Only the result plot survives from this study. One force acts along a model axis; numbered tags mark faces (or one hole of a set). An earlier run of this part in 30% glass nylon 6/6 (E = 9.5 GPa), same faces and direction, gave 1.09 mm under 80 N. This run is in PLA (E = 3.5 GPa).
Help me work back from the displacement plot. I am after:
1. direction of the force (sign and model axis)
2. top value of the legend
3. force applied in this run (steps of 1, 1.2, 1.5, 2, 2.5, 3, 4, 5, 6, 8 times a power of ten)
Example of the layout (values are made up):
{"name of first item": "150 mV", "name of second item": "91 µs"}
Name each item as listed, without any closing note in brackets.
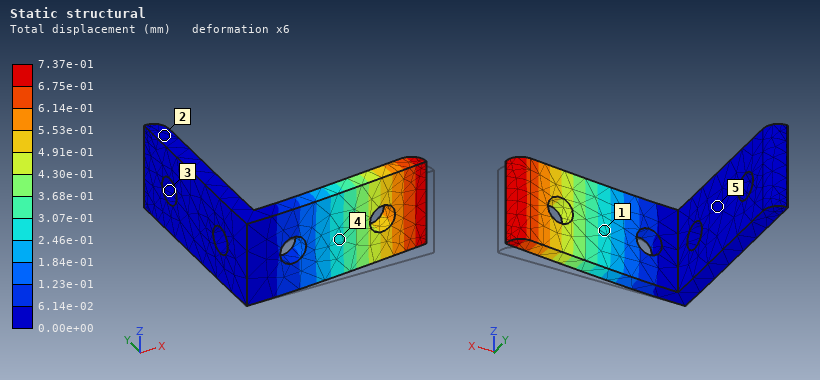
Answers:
{"direction of the force": "+Y", "top value of the legend": "7.37e-01 mm", "force applied in this run": "20 N"}
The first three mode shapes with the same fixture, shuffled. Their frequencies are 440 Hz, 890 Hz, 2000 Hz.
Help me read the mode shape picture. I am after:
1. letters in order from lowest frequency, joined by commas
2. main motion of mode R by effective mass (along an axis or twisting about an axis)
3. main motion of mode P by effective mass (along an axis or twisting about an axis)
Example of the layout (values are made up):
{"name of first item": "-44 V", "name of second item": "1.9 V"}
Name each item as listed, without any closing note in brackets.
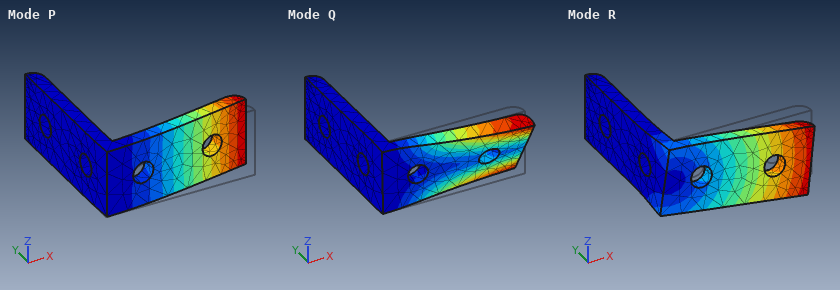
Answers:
{"letters in order from lowest frequency, joined by commas": "P, R, Q", "main motion of mode R by effective mass": "along Z", "main motion of mode P by effective mass": "along Y"}
